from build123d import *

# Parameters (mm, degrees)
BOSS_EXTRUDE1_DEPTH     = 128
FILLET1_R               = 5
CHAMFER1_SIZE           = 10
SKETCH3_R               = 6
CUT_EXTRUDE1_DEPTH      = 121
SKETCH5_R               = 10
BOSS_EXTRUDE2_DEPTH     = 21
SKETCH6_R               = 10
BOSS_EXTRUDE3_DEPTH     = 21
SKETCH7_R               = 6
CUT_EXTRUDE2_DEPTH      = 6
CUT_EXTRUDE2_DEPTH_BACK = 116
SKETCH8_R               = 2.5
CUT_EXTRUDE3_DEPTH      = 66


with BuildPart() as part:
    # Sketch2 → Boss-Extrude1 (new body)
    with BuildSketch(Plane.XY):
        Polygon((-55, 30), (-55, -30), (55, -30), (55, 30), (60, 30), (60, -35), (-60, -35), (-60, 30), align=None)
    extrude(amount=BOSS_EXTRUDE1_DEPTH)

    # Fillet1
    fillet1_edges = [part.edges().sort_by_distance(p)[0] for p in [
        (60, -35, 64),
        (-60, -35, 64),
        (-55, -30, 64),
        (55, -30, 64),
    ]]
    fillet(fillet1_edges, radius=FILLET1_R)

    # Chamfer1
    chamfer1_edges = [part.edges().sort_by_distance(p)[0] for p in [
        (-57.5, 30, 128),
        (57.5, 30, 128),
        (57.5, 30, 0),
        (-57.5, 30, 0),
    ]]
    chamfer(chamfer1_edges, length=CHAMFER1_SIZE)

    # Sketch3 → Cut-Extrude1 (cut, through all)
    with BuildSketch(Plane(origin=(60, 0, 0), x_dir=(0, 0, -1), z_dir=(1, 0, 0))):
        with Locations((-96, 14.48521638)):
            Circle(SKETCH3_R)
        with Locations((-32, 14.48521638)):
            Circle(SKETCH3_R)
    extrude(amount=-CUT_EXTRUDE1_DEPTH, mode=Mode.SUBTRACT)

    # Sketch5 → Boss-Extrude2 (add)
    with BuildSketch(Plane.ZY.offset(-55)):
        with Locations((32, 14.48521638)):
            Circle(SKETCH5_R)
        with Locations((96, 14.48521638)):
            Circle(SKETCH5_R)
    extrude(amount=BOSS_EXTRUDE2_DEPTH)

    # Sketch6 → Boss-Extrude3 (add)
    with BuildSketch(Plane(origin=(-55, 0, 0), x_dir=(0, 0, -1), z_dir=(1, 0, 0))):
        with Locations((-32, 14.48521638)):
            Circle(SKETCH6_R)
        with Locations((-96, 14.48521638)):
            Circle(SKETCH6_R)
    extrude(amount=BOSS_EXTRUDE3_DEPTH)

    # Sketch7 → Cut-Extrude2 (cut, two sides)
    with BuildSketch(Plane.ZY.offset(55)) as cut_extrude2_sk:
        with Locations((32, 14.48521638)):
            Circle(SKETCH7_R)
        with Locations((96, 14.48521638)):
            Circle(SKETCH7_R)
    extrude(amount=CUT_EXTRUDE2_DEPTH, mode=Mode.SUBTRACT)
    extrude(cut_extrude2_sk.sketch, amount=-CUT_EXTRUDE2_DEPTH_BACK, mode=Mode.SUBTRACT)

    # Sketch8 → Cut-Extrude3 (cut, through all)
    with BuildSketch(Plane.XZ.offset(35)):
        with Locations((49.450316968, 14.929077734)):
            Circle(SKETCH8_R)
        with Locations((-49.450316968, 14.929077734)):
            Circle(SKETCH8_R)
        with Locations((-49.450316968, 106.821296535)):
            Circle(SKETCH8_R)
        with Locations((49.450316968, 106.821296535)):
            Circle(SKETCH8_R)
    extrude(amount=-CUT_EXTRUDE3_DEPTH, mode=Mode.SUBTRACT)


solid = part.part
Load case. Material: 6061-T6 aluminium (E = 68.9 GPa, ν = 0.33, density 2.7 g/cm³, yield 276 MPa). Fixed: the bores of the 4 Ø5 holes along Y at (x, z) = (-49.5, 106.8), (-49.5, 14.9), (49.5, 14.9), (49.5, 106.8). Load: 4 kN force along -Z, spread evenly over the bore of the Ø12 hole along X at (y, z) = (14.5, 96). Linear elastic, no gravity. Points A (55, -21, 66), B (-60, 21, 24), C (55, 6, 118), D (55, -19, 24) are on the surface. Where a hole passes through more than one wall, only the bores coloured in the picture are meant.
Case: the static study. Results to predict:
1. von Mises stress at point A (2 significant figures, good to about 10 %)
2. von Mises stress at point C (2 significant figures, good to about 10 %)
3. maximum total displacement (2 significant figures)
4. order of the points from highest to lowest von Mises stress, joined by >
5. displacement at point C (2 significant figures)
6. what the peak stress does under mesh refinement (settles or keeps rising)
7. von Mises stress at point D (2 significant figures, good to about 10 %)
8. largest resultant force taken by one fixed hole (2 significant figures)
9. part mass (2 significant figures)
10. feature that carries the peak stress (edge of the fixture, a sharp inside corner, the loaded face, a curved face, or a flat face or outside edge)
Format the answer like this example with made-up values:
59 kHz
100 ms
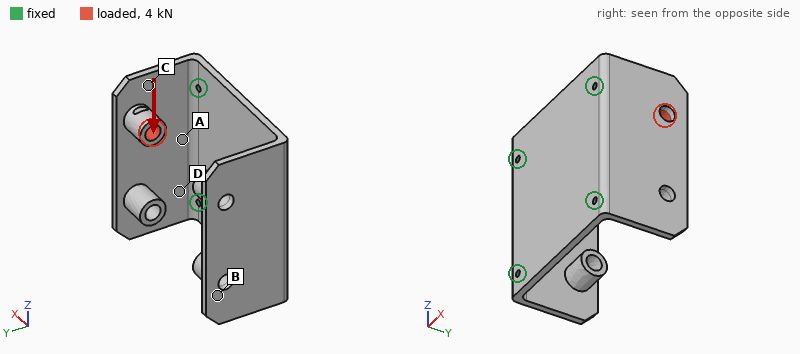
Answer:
42 MPa
78 MPa
0.75 mm
C > A > D > B
0.45 mm
keeps rising
23 MPa
2.9 kN
450 g
edge of the fixture
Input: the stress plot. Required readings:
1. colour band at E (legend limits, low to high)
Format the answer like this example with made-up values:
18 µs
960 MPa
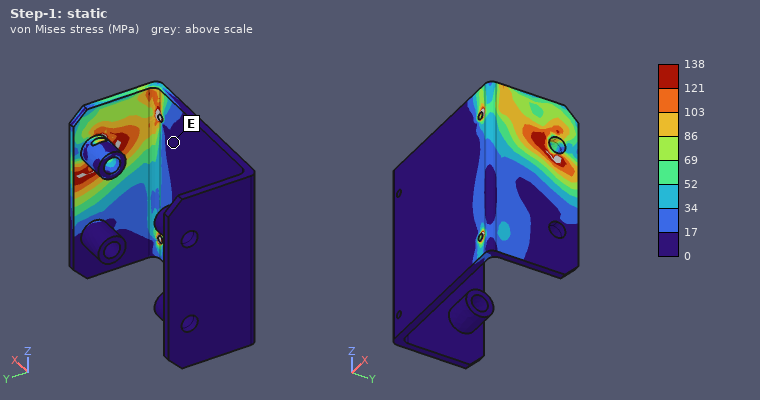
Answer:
0 to 17 MPa
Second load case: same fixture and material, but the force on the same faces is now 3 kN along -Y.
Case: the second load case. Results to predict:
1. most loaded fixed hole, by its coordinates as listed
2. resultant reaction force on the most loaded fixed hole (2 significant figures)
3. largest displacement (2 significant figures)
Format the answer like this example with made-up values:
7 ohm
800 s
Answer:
(49.5, 106.8)
2.6 kN
1.1 mm
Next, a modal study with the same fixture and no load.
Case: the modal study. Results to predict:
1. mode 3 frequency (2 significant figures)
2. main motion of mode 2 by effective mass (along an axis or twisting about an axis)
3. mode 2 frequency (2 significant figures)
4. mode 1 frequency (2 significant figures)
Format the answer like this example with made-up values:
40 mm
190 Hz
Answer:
1400 Hz
along X
790 Hz
760 Hz
